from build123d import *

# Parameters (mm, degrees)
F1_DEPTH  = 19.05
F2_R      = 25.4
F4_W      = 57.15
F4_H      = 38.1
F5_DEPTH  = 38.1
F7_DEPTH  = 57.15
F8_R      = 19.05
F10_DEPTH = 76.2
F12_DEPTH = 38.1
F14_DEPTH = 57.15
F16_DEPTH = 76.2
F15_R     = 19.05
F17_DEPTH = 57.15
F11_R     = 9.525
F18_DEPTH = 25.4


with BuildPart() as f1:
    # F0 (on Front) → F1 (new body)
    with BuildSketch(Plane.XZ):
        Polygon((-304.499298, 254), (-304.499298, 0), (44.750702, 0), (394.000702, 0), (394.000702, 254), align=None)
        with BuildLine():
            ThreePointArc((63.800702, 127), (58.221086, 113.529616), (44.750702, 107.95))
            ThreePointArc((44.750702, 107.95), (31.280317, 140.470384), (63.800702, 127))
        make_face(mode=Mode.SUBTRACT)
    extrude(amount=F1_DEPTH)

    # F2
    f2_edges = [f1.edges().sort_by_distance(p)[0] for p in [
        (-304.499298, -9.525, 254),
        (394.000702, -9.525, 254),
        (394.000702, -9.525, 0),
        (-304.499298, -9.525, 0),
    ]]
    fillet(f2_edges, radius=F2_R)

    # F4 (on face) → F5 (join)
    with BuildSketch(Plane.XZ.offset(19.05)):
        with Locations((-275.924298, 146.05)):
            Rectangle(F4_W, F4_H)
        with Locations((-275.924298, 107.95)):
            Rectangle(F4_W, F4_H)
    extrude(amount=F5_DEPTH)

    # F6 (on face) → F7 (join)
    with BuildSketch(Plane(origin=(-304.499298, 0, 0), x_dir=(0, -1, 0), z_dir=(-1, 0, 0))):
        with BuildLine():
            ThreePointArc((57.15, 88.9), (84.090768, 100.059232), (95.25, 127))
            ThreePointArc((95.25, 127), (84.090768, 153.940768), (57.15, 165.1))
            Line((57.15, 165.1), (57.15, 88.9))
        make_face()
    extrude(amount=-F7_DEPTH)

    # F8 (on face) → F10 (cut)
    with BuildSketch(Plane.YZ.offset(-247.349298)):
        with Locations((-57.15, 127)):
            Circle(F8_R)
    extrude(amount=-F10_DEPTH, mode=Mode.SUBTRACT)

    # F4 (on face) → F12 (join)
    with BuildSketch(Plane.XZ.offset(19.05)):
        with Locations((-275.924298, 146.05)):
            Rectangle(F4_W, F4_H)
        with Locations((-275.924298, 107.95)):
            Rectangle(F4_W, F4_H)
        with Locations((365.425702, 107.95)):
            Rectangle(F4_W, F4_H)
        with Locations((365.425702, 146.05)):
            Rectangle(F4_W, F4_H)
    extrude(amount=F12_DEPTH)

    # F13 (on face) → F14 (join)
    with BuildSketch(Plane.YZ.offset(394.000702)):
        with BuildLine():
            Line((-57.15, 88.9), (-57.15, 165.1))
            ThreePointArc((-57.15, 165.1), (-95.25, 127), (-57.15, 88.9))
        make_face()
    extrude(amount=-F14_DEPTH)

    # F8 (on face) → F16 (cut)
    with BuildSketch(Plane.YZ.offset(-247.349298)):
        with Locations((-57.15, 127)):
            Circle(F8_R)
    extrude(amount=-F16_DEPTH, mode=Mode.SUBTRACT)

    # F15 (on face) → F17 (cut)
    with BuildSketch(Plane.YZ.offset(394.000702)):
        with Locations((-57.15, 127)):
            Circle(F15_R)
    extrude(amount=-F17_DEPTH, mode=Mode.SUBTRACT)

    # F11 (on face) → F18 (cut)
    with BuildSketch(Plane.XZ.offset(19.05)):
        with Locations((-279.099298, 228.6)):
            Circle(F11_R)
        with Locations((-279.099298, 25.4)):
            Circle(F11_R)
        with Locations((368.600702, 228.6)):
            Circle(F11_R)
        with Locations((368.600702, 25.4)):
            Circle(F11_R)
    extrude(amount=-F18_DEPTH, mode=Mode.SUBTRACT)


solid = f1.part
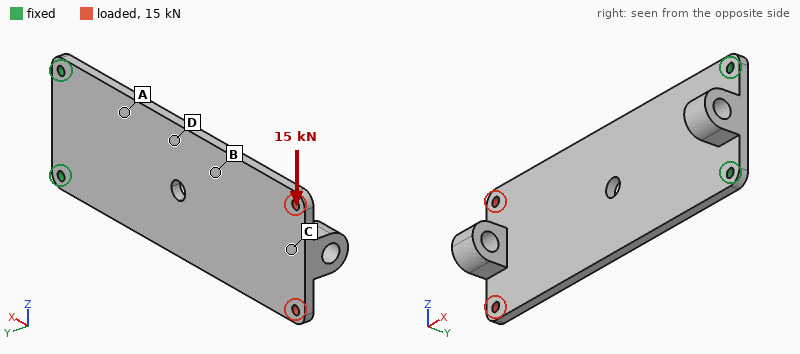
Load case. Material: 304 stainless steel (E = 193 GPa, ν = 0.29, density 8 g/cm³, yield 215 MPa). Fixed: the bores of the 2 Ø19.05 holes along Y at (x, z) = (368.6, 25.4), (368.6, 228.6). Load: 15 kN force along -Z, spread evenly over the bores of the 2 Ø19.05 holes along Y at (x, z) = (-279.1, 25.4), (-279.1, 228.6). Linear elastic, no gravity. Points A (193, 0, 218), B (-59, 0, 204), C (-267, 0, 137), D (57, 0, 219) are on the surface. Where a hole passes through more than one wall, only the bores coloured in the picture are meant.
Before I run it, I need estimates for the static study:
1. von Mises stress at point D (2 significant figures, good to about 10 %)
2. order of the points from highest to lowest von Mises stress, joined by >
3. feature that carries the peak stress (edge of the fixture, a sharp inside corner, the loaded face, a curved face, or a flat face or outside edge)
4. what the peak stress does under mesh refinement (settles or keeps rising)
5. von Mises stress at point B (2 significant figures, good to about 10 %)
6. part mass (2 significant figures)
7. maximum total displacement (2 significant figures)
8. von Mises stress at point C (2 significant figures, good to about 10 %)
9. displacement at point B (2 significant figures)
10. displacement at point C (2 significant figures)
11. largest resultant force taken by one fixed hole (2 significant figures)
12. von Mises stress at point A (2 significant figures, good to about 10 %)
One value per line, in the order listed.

19 MPa
A > D > B > C
edge of the fixture
keeps rising
11 MPa
30 kg
0.34 mm
5.5 MPa
0.17 mm
0.31 mm
48 kN
25 MPa
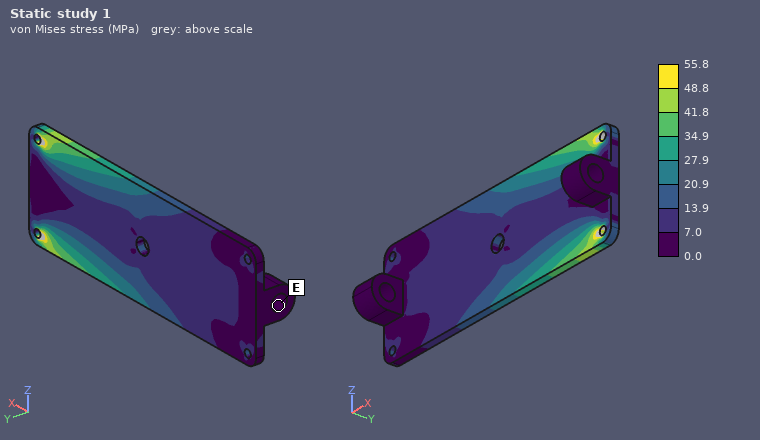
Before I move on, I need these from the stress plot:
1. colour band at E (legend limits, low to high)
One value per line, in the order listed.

0.0 to 7.0 MPa
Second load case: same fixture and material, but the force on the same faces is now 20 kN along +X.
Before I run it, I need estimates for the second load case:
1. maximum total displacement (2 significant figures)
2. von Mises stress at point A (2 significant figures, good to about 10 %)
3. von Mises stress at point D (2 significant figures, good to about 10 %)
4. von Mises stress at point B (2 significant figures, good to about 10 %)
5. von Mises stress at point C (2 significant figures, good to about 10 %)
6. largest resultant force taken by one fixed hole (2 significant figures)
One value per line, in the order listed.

19 µm
4.3 MPa
4.2 MPa
4.3 MPa
2.0 MPa
10 kN
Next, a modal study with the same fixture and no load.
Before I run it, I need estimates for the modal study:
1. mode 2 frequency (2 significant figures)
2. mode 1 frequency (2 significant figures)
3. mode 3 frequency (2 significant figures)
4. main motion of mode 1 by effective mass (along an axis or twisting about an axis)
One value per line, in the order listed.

180 Hz
29 Hz
190 Hz
along Y
